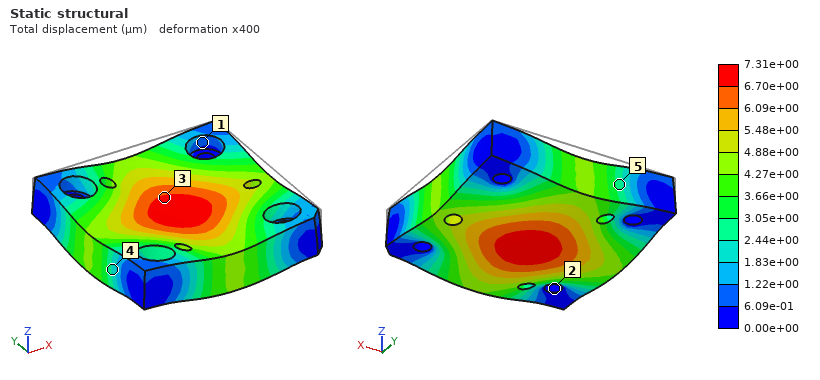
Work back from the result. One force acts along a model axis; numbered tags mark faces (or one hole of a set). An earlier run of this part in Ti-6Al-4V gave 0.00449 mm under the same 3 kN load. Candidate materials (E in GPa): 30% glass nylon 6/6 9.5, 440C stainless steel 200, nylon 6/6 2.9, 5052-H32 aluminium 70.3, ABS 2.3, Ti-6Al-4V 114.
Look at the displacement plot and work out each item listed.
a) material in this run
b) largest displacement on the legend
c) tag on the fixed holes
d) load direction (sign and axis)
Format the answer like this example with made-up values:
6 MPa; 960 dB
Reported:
5052-H32 aluminium; 7.31e+00 µm; 2; -Z
